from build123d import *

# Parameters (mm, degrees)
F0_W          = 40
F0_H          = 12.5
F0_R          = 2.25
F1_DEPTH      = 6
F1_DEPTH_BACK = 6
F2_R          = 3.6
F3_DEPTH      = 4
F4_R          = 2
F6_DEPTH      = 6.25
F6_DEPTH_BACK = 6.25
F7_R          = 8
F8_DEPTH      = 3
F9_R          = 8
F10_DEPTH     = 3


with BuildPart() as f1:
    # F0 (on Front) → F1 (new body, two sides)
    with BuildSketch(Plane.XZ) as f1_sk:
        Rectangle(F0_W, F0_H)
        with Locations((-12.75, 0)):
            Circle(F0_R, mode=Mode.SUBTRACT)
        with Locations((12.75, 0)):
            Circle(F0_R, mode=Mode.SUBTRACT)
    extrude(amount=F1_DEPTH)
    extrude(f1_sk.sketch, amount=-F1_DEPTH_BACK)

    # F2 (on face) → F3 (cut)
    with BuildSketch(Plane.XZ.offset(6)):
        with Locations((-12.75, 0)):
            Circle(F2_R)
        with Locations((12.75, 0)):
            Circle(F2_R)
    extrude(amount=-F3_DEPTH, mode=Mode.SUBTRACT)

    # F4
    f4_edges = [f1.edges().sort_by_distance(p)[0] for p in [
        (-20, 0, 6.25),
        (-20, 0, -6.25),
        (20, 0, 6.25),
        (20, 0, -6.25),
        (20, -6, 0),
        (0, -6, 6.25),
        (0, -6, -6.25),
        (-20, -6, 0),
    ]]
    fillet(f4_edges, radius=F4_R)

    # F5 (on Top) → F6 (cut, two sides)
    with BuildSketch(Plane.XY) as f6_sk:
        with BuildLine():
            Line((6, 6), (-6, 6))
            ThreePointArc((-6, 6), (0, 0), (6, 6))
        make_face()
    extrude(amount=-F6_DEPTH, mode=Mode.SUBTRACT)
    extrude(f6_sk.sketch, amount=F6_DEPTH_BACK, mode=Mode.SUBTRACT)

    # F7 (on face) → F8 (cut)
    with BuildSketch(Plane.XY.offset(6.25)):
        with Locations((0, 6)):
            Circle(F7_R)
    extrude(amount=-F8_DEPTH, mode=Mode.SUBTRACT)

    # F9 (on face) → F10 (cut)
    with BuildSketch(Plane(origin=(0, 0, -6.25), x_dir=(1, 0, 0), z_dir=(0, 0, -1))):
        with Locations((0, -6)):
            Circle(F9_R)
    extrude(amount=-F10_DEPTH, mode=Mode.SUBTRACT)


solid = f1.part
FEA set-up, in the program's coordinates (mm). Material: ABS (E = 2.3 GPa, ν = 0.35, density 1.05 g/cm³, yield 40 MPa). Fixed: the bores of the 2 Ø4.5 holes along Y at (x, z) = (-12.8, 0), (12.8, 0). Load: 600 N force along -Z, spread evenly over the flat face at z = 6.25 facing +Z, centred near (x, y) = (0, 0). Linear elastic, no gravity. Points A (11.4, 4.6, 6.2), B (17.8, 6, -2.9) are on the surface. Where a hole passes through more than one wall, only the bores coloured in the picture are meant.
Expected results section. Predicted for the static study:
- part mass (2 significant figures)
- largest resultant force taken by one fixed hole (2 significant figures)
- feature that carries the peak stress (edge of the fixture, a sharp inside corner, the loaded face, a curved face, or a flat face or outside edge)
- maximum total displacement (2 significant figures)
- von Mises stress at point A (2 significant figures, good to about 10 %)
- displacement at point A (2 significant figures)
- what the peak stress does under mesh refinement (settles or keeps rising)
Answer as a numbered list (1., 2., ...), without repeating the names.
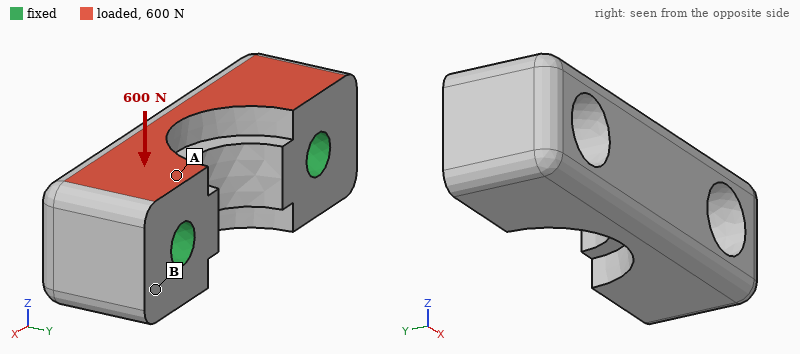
1. 4.5 g
2. 300 N
3. edge of the fixture
4. 27 µm
5. 3.3 MPa
6. 7.3 µm
7. keeps rising
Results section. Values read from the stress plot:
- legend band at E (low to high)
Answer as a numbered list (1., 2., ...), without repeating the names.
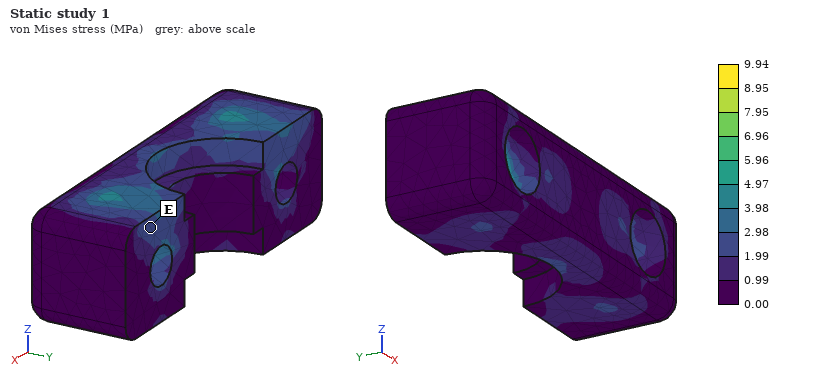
1. 1.99 to 2.98 MPa
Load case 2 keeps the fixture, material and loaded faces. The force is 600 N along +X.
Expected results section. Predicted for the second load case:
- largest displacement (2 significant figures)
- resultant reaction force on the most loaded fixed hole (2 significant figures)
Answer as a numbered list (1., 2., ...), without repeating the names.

1. 29 µm
2. 310 N
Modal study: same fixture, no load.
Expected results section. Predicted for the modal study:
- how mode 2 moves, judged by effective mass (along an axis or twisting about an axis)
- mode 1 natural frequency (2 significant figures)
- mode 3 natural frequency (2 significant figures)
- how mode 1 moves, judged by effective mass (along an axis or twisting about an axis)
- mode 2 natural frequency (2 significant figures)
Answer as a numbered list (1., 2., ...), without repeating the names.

1. along Y
2. 11 kHz
3. 17 kHz
4. along Z
5. 16 kHz
